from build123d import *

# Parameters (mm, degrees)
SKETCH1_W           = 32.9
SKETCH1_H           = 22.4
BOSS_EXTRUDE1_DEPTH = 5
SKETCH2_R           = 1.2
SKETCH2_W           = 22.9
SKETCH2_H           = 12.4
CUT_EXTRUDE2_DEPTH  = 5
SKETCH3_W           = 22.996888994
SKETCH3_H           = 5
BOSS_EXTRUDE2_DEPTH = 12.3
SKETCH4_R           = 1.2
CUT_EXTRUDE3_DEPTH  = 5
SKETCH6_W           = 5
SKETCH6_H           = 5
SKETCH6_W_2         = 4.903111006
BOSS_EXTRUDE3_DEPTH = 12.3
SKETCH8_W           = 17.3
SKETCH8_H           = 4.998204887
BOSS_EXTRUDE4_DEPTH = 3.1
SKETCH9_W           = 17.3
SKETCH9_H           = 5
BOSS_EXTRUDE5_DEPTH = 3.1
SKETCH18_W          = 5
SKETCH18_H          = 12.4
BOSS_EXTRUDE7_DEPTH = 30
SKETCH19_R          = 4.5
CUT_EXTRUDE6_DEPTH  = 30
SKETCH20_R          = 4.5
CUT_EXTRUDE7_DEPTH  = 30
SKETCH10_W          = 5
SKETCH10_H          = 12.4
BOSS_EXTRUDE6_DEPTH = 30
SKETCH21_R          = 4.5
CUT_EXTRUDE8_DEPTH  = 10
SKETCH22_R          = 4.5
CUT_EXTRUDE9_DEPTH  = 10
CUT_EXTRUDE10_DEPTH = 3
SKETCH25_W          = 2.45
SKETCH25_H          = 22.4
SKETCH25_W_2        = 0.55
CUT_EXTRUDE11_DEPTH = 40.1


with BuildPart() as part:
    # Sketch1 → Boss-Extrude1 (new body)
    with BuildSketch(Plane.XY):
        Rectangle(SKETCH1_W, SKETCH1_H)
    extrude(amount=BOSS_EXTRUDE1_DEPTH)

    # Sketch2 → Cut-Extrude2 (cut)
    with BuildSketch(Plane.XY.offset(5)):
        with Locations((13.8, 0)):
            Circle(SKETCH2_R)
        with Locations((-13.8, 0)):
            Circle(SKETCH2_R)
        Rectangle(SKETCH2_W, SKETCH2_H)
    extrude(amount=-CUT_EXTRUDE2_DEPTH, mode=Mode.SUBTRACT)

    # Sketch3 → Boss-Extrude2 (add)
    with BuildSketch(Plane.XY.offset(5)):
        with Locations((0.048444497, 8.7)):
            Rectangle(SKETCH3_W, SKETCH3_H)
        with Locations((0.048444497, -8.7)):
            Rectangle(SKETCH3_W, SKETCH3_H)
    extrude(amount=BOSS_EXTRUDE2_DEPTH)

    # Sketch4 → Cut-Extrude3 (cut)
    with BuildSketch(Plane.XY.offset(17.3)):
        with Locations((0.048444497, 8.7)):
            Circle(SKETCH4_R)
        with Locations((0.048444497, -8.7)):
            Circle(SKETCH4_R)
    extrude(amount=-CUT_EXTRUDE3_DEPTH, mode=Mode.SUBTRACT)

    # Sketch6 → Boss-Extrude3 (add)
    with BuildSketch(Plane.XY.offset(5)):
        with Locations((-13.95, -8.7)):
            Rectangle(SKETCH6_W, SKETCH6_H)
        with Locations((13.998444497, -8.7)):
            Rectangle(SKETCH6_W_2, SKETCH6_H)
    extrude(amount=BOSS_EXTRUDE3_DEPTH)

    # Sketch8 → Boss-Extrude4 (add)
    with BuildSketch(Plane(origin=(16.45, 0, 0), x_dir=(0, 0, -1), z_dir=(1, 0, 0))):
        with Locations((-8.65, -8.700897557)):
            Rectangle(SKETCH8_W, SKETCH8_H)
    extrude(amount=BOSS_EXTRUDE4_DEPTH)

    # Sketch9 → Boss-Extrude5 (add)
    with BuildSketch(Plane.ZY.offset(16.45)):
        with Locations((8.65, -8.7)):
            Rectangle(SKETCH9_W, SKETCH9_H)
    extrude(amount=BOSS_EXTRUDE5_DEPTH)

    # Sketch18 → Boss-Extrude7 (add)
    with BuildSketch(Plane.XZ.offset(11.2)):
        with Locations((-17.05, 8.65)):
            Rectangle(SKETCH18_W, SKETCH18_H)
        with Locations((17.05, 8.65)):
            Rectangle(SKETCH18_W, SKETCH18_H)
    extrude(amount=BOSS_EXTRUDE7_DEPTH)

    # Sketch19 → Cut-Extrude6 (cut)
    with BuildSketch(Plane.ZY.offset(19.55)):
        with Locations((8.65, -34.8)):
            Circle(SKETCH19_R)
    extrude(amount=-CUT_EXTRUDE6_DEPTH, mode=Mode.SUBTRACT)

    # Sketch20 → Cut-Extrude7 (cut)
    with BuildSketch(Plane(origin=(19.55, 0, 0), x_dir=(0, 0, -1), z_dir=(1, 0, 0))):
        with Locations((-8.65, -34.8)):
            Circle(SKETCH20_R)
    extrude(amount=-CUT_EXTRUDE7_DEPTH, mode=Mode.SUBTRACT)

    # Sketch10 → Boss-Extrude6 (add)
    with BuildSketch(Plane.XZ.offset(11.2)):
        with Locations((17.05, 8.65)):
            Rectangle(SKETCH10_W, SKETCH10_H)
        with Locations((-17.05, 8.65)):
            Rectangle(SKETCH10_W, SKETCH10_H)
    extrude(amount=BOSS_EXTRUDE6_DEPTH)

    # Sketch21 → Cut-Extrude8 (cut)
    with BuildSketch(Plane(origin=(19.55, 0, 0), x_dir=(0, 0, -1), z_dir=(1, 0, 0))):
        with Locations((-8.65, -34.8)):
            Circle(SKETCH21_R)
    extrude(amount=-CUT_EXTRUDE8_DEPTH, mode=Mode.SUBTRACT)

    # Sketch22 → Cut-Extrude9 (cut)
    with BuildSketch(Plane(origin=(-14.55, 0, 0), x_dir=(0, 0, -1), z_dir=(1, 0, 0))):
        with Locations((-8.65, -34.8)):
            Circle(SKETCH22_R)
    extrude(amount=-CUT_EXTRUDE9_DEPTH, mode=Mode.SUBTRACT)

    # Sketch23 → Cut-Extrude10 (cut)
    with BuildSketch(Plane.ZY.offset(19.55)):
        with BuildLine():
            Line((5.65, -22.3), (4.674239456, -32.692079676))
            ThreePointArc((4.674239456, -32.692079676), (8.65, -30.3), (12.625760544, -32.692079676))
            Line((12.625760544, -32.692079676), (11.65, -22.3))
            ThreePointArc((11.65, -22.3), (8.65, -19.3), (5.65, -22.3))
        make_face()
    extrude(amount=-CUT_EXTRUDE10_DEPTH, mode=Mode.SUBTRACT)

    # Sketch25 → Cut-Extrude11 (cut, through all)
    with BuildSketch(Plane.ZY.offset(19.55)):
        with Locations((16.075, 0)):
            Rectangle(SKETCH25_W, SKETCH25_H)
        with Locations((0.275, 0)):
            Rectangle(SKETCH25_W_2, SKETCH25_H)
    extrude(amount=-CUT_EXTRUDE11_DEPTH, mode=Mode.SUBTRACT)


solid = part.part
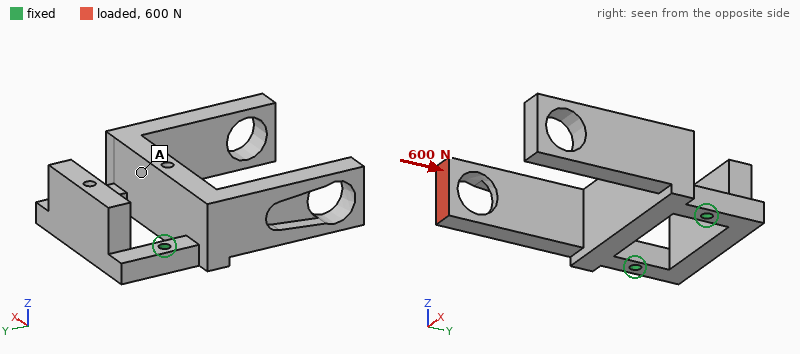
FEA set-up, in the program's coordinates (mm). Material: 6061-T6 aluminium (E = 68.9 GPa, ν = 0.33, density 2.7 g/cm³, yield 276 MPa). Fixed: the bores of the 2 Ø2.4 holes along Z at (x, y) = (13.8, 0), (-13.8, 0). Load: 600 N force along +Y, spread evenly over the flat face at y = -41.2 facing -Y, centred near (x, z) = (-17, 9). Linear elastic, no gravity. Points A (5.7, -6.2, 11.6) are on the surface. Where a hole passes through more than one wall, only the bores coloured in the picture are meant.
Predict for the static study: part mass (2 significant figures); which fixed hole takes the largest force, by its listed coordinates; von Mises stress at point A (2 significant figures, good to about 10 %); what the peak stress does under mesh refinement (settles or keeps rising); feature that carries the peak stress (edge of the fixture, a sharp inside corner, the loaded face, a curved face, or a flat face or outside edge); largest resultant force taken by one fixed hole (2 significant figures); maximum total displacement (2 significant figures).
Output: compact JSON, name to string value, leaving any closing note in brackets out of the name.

{"part mass": "22 g", "which fixed hole takes the largest force, by its listed coordinates": "(-13.8, 0)", "von Mises stress at point A": "19 MPa", "what the peak stress does under mesh refinement": "keeps rising", "feature that carries the peak stress": "edge of the fixture", "largest resultant force taken by one fixed hole": "660 N", "maximum total displacement": "0.27 mm"}
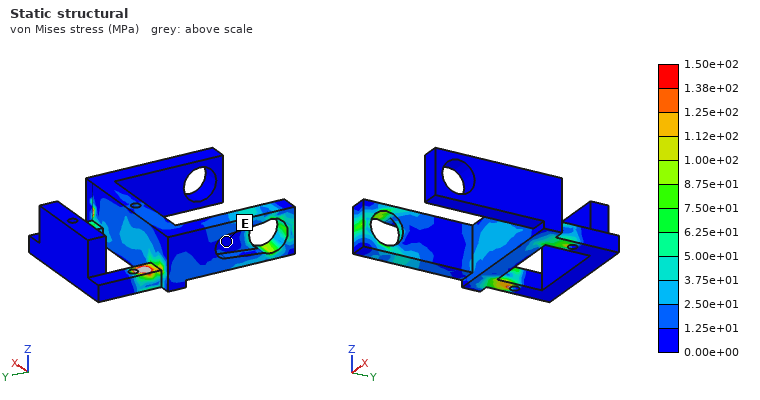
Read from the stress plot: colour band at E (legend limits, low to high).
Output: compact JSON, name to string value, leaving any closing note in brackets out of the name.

{"colour band at E": "0.00e+00 to 1.25e+01 MPa"}
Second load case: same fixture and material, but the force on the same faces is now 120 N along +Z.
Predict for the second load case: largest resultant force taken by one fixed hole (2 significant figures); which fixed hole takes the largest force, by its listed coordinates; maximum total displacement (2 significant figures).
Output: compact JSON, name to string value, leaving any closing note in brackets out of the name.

{"largest resultant force taken by one fixed hole": "120 N", "which fixed hole takes the largest force, by its listed coordinates": "(-13.8, 0)", "maximum total displacement": "0.39 mm"}
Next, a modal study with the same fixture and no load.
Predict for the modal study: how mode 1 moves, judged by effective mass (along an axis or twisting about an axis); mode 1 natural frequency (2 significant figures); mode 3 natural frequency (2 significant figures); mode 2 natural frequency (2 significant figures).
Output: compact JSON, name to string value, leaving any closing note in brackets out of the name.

{"how mode 1 moves, judged by effective mass": "along Z", "mode 1 natural frequency": "1900 Hz", "mode 3 natural frequency": "3600 Hz", "mode 2 natural frequency": "3100 Hz"}
